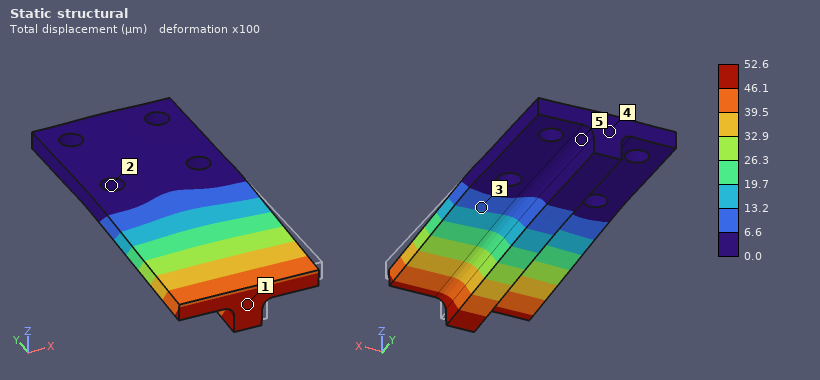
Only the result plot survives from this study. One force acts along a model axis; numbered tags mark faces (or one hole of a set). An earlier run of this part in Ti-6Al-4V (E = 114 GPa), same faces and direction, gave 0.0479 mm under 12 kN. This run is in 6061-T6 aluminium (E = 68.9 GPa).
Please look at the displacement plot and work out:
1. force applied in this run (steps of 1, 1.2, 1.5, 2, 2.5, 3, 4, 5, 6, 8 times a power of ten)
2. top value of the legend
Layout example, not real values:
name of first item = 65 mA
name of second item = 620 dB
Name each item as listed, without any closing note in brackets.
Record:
force applied in this run = 8 kN
top value of the legend = 52.6 µm
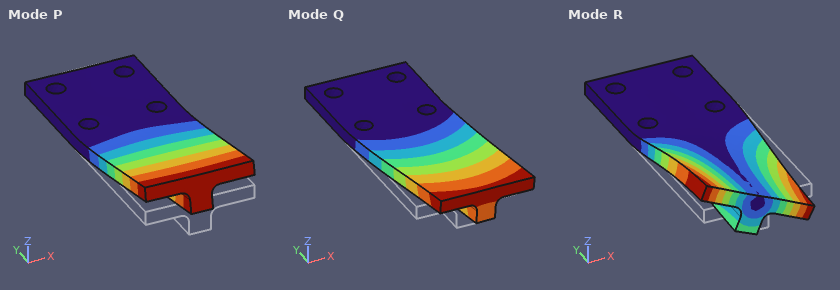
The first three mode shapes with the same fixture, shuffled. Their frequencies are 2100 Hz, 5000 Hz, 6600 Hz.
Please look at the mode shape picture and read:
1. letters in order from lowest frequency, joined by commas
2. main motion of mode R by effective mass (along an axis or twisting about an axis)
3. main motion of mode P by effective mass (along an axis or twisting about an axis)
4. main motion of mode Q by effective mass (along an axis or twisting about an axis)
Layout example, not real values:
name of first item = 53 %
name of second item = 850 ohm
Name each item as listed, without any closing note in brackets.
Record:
letters in order from lowest frequency, joined by commas = P, R, Q
main motion of mode R by effective mass = twisting about Y
main motion of mode P by effective mass = along Z
main motion of mode Q by effective mass = along X
